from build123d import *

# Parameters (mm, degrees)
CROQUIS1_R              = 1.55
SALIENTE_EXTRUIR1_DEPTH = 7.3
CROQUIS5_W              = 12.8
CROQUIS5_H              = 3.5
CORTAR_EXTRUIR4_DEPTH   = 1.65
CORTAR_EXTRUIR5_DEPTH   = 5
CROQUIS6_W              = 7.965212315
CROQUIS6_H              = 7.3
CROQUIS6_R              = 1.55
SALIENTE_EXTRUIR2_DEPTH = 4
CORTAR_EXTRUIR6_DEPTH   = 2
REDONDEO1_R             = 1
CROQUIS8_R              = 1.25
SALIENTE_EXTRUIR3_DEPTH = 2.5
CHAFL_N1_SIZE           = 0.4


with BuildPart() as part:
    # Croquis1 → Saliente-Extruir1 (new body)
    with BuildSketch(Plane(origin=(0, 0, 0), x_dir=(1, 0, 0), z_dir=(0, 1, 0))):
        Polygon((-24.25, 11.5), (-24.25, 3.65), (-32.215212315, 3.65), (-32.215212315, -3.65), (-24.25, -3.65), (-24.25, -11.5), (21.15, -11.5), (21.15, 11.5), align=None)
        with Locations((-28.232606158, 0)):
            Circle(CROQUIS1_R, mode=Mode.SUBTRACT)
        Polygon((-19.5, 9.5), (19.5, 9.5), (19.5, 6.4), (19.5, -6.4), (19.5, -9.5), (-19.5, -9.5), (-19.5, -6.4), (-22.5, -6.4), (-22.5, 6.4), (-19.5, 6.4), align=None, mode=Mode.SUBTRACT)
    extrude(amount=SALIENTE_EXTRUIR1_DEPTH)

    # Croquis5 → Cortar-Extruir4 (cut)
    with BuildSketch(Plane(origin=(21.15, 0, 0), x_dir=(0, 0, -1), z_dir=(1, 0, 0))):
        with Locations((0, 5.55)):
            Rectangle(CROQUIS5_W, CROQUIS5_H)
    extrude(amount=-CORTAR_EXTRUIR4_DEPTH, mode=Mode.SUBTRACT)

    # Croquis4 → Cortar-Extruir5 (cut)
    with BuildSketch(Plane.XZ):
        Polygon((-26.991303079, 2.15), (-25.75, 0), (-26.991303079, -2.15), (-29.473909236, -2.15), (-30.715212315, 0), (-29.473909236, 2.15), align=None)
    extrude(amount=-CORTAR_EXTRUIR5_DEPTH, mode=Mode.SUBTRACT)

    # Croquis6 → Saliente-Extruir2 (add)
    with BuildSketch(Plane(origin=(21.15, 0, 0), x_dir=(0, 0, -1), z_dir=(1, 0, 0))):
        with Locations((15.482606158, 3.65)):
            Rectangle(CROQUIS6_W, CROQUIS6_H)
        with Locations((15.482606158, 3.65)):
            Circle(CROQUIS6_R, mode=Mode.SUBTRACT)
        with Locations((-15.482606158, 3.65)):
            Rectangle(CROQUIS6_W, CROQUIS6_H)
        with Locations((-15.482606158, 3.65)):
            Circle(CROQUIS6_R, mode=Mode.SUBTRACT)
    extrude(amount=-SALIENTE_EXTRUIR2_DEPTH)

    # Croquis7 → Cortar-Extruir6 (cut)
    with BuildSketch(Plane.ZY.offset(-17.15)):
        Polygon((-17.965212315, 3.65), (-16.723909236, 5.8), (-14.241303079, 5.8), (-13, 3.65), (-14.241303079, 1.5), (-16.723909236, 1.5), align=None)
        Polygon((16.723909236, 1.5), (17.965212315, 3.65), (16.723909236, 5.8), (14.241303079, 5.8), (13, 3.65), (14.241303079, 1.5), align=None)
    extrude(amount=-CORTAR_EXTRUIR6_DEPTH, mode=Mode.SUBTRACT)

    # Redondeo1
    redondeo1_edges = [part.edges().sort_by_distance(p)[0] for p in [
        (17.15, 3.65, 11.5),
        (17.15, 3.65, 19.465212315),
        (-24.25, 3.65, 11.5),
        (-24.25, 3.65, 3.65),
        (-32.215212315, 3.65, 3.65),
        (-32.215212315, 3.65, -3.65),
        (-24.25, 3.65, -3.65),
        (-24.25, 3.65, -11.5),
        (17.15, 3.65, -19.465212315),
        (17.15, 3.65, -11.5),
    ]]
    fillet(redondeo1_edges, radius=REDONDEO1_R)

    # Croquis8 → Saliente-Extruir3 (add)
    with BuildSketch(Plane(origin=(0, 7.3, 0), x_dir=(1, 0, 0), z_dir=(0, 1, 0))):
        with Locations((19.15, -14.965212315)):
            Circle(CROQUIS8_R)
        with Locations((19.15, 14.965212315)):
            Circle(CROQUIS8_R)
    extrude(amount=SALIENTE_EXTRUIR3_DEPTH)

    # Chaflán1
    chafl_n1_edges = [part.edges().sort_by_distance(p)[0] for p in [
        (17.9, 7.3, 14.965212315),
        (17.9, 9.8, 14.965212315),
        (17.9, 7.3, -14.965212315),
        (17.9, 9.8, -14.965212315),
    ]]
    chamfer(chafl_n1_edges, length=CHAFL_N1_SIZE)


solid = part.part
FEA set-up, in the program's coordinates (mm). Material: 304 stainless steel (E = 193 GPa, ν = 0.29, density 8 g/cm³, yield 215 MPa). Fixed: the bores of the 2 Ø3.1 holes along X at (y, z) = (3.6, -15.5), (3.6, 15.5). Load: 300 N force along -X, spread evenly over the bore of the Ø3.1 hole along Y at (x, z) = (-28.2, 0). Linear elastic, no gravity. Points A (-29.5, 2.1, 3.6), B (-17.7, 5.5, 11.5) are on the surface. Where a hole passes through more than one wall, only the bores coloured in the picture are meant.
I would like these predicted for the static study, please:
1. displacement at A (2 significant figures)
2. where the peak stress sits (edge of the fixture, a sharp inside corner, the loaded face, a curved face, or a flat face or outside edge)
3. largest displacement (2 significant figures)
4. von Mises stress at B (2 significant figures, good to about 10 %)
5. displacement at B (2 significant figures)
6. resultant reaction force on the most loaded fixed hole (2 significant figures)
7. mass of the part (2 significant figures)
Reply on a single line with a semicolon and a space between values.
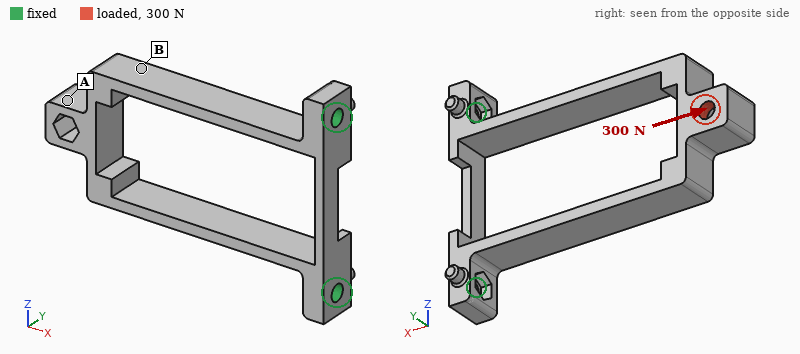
58 µm; a curved face; 69 µm; 39 MPa; 35 µm; 150 N; 21 g
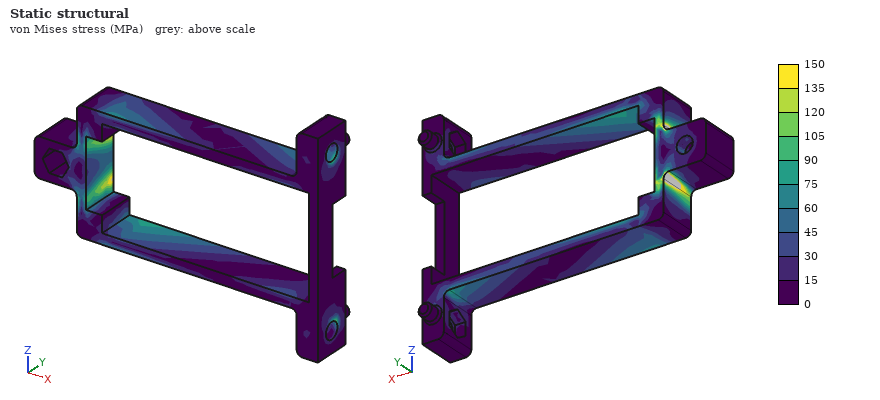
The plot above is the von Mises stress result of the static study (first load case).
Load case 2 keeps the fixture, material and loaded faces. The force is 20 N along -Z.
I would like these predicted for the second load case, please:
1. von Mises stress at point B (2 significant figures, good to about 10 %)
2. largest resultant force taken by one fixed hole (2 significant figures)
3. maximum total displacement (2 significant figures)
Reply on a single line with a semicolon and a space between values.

29 MPa; 28 N; 59 µm
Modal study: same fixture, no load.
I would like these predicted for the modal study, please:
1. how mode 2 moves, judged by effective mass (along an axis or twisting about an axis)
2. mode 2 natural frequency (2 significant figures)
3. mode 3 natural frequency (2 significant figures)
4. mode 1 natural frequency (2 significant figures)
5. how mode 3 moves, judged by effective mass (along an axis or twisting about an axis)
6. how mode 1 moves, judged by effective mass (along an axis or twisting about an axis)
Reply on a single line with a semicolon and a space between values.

along Y; 1200 Hz; 2900 Hz; 950 Hz; twisting about X; along Z
